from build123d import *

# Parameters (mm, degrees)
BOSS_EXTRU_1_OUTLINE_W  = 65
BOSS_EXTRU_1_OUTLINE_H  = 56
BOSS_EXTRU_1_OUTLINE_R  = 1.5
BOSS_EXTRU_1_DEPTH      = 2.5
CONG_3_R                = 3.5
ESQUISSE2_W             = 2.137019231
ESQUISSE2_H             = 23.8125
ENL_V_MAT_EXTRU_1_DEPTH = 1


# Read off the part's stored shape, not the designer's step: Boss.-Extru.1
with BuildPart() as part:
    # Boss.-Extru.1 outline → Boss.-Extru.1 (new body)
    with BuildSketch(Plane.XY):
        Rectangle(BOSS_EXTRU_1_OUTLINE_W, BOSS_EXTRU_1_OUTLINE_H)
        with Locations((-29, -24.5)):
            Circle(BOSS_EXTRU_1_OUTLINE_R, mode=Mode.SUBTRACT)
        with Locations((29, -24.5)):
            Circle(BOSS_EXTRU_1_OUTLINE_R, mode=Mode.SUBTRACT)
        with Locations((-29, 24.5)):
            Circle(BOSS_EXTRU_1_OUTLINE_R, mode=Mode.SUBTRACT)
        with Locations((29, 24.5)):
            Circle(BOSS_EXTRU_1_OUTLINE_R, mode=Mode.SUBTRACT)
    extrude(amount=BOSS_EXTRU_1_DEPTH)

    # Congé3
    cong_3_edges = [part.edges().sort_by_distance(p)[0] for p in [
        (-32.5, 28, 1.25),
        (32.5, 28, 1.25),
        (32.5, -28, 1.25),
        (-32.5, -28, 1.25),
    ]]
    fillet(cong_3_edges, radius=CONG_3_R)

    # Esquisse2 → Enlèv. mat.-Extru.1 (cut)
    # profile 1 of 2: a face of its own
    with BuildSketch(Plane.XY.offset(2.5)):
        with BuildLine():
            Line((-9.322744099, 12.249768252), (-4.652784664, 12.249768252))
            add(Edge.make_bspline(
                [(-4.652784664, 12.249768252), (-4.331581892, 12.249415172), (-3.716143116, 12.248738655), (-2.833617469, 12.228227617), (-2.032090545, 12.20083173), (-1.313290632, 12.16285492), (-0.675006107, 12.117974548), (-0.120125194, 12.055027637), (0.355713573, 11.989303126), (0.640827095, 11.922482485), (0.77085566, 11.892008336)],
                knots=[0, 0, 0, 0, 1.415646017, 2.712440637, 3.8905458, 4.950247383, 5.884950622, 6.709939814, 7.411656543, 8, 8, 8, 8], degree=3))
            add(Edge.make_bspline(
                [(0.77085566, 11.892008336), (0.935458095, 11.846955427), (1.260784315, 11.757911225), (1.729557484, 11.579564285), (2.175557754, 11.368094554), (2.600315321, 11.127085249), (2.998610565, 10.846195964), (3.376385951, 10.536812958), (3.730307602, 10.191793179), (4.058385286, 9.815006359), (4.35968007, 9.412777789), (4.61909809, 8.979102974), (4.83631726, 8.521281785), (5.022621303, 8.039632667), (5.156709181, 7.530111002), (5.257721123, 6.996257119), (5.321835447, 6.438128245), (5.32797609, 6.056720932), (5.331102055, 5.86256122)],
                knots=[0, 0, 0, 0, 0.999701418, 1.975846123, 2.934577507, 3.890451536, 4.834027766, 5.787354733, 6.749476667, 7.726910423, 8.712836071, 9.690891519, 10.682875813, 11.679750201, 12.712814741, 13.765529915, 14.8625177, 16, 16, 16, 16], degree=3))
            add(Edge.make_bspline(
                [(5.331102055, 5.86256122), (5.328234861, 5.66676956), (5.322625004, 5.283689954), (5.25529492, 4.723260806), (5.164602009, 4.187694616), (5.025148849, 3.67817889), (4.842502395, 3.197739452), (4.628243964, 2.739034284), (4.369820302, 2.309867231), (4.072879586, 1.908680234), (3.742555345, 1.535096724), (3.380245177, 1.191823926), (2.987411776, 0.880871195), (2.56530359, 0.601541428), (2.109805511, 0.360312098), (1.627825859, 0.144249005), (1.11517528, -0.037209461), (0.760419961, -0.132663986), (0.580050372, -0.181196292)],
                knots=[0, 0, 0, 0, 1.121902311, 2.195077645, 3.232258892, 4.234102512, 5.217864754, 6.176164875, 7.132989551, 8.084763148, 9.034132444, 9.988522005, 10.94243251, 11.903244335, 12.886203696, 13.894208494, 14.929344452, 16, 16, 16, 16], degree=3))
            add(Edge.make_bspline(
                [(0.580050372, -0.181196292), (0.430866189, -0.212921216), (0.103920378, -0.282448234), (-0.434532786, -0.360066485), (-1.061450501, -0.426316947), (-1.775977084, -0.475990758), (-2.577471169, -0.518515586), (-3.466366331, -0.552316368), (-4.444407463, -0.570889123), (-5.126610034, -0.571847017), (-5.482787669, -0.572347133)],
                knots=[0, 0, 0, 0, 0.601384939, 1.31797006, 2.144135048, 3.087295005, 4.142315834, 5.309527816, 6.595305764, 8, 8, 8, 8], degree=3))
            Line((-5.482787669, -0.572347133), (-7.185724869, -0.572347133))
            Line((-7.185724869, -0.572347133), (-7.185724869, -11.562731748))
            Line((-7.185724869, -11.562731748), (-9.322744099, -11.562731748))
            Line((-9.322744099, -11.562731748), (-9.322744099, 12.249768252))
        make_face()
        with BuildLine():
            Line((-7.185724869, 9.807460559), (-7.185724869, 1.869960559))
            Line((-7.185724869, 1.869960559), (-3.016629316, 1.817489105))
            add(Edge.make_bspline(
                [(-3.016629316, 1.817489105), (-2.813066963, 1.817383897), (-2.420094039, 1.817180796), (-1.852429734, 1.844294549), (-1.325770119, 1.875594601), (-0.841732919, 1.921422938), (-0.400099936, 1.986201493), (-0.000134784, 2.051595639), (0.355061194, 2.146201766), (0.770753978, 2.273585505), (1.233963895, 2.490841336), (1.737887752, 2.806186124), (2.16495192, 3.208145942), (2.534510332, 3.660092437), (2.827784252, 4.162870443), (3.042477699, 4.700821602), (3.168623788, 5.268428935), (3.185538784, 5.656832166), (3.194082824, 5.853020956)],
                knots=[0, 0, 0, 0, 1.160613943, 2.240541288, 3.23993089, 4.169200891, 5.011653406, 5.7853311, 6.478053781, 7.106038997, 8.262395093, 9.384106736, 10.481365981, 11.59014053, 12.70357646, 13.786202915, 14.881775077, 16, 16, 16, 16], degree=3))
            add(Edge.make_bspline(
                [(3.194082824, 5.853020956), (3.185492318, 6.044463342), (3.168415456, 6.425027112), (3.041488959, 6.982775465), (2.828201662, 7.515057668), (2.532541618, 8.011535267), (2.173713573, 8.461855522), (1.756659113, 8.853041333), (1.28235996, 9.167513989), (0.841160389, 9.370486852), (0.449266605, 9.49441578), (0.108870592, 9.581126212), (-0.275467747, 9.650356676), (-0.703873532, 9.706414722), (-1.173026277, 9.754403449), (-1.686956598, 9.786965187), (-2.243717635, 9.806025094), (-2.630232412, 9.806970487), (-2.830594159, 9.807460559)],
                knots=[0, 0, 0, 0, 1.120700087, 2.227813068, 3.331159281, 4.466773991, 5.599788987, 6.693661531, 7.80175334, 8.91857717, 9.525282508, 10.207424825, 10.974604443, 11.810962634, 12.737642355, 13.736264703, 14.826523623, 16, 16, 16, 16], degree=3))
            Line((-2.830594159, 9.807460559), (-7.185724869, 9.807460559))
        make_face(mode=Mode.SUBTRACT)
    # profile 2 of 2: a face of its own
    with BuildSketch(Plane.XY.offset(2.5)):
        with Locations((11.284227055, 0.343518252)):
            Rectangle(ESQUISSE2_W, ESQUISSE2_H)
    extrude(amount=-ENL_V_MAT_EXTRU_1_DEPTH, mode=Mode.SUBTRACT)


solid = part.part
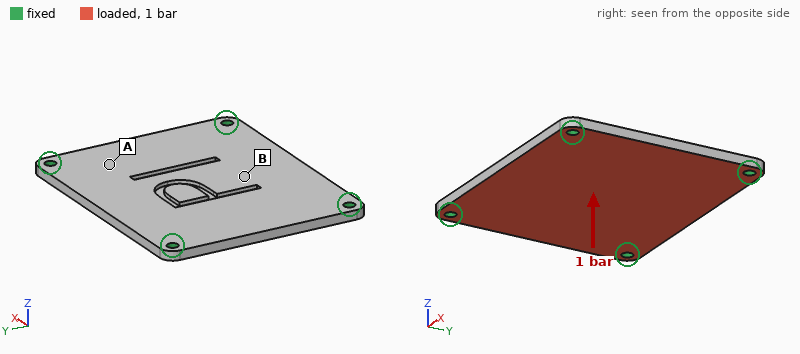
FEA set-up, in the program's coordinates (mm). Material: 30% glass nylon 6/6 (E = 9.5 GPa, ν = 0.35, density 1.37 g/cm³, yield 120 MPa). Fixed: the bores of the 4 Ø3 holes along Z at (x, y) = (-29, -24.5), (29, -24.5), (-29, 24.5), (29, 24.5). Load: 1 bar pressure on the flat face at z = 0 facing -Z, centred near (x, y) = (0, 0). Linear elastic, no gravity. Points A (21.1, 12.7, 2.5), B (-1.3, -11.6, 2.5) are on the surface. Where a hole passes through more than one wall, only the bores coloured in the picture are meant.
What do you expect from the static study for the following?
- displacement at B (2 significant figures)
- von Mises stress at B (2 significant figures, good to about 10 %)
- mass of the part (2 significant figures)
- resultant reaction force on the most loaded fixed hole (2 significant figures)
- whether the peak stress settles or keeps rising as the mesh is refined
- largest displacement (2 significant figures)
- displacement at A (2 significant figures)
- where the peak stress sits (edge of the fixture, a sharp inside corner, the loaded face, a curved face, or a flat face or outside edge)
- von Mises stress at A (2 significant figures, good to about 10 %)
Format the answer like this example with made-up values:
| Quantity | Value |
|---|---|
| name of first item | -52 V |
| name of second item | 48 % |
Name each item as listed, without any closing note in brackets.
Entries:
| Quantity | Value |
|---|---|
| displacement at B | 0.48 mm |
| von Mises stress at B | 15 MPa |
| mass of the part | 12 g |
| resultant reaction force on the most loaded fixed hole | 94 N |
| whether the peak stress settles or keeps rising as the mesh is refined | keeps rising |
| largest displacement | 0.56 mm |
| displacement at A | 0.23 mm |
| where the peak stress sits | edge of the fixture |
| von Mises stress at A | 6.4 MPa |
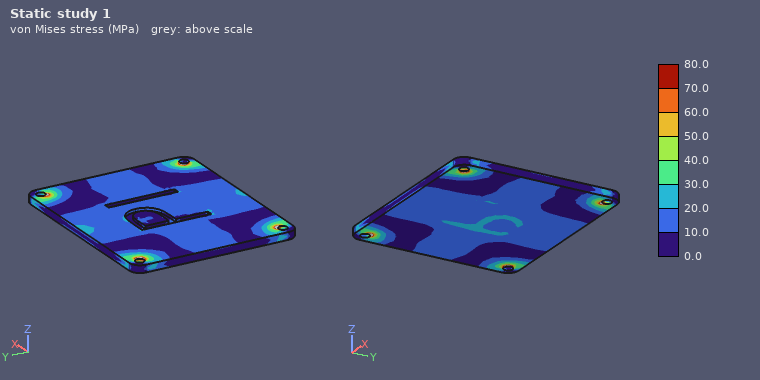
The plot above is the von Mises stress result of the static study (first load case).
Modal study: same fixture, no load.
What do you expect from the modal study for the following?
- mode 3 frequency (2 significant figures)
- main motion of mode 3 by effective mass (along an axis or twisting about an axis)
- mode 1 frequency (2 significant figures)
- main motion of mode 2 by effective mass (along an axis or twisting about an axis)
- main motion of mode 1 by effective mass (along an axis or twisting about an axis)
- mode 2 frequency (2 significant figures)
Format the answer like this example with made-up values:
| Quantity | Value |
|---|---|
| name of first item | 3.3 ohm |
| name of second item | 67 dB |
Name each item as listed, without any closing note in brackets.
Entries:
| Quantity | Value |
|---|---|
| mode 3 frequency | 2900 Hz |
| main motion of mode 3 by effective mass | twisting about Y |
| mode 1 frequency | 1400 Hz |
| main motion of mode 2 by effective mass | twisting about X |
| main motion of mode 1 by effective mass | along Z |
| mode 2 frequency | 2400 Hz |
